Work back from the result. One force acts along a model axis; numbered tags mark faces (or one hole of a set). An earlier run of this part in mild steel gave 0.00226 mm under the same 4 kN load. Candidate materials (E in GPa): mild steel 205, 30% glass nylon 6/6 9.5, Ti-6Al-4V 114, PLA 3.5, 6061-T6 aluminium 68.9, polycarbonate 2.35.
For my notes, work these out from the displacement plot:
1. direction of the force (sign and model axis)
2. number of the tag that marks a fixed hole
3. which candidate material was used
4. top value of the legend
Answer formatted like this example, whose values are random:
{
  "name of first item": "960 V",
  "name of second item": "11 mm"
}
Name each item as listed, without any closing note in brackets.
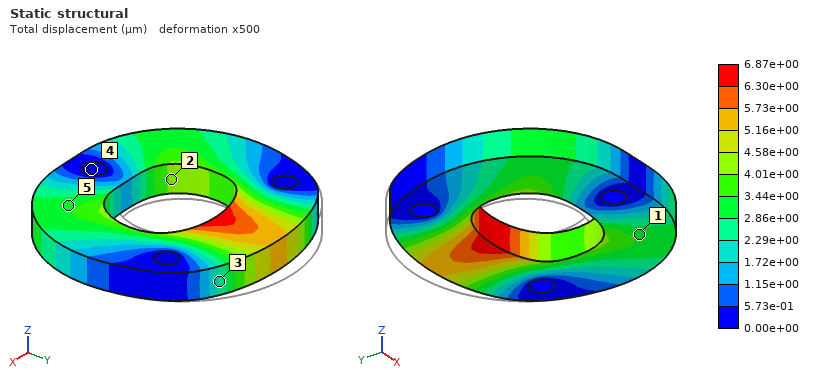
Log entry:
{
  "direction of the force": "-Y",
  "number of the tag that marks a fixed hole": "4",
  "which candidate material was used": "6061-T6 aluminium",
  "top value of the legend": "6.87e+00 µm"
}
